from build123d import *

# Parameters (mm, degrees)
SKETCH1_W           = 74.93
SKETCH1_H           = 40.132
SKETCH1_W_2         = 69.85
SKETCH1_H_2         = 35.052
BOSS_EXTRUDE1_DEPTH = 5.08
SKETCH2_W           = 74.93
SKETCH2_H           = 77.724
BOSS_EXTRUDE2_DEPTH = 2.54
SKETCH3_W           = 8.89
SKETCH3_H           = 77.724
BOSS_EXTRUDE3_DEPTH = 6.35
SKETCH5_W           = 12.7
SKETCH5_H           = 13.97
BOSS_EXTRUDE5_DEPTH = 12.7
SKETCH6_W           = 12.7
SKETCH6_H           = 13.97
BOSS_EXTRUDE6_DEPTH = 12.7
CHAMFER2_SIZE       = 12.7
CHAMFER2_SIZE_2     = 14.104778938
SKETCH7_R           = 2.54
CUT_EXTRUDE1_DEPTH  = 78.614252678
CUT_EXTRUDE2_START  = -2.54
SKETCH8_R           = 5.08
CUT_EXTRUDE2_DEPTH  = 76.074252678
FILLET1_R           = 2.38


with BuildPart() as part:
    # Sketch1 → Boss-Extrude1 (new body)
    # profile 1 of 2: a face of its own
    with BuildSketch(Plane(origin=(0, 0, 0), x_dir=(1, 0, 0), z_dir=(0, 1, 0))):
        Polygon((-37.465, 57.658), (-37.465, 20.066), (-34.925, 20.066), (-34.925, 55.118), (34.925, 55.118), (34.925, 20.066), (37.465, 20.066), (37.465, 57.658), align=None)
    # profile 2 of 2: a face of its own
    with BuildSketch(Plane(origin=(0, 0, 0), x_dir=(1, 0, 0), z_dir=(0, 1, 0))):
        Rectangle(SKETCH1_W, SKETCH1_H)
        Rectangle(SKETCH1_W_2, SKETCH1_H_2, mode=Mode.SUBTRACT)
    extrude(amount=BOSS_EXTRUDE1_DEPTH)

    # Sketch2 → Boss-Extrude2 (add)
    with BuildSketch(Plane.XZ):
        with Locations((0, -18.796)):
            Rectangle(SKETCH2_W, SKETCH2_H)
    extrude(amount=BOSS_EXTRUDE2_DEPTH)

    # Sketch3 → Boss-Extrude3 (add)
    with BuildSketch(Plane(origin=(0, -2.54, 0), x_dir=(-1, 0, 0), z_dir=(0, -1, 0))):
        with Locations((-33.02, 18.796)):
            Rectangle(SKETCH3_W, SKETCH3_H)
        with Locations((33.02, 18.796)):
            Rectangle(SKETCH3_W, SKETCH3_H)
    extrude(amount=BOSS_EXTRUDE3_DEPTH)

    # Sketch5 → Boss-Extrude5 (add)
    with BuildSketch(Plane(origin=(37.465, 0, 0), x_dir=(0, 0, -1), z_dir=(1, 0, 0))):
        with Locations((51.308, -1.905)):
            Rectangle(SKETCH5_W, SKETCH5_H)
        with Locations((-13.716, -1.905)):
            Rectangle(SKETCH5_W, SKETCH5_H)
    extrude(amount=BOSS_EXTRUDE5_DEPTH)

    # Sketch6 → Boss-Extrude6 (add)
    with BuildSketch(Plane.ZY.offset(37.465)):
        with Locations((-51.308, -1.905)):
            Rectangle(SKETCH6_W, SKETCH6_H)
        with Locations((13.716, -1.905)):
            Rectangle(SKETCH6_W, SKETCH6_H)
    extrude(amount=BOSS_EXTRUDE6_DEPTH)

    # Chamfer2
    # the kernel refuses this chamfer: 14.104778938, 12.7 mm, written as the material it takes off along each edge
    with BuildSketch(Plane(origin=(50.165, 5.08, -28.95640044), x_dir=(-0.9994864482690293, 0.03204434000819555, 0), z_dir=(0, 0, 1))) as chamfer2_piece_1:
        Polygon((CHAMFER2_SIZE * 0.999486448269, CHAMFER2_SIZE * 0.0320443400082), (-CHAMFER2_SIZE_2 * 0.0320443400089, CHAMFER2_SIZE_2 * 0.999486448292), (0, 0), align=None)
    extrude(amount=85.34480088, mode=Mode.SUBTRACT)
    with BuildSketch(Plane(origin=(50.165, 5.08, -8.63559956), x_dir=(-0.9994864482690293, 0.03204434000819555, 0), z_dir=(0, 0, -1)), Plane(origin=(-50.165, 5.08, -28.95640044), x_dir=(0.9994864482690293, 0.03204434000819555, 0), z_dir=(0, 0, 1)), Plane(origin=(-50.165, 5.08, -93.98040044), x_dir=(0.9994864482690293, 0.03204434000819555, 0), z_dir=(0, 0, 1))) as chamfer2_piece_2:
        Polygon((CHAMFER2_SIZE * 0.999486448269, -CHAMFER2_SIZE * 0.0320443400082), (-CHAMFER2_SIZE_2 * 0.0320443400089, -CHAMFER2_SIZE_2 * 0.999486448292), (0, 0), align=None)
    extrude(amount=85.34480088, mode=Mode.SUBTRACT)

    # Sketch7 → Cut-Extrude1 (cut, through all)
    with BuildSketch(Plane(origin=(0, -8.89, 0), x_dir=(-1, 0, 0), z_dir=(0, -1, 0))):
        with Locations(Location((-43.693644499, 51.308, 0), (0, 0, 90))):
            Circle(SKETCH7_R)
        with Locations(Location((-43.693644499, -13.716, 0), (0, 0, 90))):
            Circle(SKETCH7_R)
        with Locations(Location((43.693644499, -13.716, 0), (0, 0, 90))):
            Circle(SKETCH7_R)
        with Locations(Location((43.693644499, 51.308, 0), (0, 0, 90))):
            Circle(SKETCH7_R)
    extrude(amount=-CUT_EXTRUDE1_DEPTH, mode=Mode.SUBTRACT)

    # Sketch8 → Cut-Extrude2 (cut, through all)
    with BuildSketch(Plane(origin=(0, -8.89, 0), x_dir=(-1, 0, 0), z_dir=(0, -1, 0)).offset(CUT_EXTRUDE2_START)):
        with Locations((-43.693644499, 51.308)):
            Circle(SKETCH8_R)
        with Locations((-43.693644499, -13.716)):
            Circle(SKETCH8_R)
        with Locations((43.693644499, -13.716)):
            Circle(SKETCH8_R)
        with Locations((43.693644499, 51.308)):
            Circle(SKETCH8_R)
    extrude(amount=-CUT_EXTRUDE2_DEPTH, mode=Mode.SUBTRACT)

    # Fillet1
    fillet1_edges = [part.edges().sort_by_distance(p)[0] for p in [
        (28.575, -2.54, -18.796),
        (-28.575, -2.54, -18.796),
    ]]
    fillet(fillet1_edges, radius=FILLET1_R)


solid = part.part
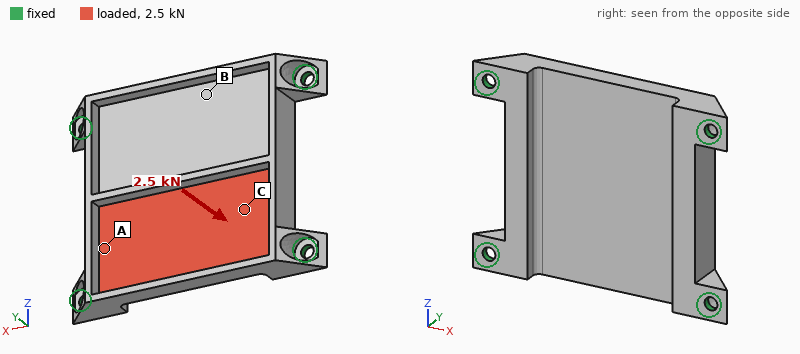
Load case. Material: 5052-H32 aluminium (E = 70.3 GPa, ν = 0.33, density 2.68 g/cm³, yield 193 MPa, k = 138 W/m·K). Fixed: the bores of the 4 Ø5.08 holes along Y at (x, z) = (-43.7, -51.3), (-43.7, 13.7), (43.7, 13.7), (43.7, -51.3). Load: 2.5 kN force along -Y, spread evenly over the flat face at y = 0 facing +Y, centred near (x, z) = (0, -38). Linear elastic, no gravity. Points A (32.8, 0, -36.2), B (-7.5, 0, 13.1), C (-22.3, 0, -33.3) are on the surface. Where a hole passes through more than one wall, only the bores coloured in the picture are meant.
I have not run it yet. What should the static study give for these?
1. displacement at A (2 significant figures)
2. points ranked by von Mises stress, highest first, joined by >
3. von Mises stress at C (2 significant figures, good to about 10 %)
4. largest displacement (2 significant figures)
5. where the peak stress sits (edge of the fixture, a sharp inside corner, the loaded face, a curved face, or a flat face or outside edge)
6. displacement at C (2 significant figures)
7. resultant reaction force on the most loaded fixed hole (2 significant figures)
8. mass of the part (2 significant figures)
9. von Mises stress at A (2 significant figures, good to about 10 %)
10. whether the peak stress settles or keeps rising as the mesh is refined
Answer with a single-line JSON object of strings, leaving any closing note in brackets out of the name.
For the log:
{"displacement at A": "0.040 mm", "points ranked by von Mises stress, highest first, joined by >": "C > A > B", "von Mises stress at C": "37 MPa", "largest displacement": "0.20 mm", "where the peak stress sits": "edge of the fixture", "displacement at C": "0.092 mm", "resultant reaction force on the most loaded fixed hole": "2.4 kN", "mass of the part": "84 g", "von Mises stress at A": "18 MPa", "whether the peak stress settles or keeps rising as the mesh is refined": "keeps rising"}
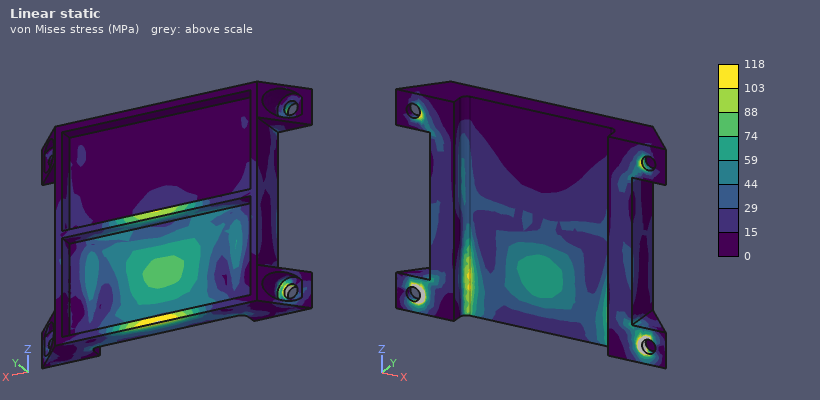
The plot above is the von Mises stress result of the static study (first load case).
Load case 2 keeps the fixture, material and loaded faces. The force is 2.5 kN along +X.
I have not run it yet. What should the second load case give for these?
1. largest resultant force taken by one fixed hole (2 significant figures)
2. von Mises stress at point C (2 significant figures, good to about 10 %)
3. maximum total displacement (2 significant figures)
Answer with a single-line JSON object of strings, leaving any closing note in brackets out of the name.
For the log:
{"largest resultant force taken by one fixed hole": "860 N", "von Mises stress at point C": "12 MPa", "maximum total displacement": "27 µm"}
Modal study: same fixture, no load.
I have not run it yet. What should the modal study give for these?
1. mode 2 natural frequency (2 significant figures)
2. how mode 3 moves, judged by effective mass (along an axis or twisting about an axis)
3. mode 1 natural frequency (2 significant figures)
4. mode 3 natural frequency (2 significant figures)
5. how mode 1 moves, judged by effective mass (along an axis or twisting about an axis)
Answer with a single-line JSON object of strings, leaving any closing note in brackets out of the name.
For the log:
{"mode 2 natural frequency": "5100 Hz", "how mode 3 moves, judged by effective mass": "twisting about X", "mode 1 natural frequency": "3900 Hz", "mode 3 natural frequency": "5500 Hz", "how mode 1 moves, judged by effective mass": "along Y"}
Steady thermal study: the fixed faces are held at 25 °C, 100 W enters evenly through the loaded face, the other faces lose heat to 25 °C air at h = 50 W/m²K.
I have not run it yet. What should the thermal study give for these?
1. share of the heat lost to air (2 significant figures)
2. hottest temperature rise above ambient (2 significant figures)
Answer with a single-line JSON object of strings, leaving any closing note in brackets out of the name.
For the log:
{"share of the heat lost to air": "25 %", "hottest temperature rise above ambient": "62 K"}
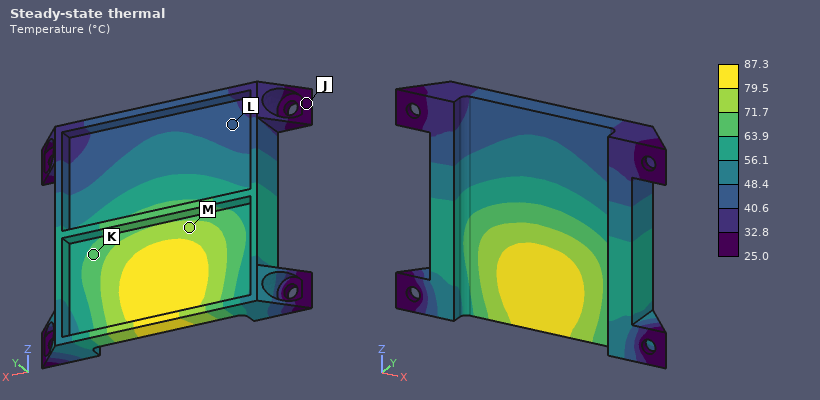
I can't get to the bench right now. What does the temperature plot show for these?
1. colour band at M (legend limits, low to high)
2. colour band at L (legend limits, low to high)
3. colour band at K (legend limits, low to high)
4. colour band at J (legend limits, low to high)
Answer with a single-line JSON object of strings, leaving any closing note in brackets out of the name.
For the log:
{"colour band at M": "71.7 to 79.5 °C", "colour band at L": "40.6 to 48.4 °C", "colour band at K": "63.9 to 71.7 °C", "colour band at J": "25.0 to 32.8 °C"}
